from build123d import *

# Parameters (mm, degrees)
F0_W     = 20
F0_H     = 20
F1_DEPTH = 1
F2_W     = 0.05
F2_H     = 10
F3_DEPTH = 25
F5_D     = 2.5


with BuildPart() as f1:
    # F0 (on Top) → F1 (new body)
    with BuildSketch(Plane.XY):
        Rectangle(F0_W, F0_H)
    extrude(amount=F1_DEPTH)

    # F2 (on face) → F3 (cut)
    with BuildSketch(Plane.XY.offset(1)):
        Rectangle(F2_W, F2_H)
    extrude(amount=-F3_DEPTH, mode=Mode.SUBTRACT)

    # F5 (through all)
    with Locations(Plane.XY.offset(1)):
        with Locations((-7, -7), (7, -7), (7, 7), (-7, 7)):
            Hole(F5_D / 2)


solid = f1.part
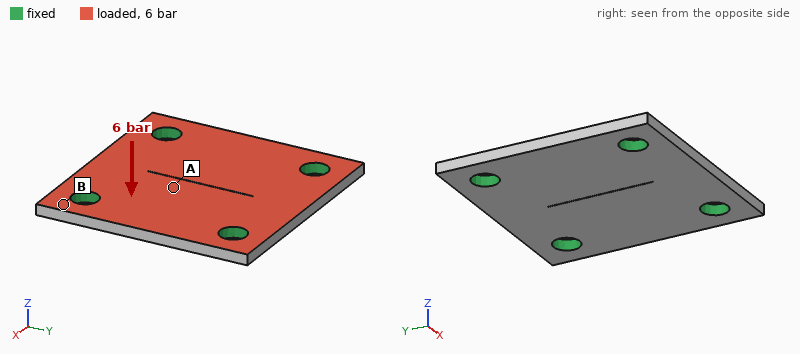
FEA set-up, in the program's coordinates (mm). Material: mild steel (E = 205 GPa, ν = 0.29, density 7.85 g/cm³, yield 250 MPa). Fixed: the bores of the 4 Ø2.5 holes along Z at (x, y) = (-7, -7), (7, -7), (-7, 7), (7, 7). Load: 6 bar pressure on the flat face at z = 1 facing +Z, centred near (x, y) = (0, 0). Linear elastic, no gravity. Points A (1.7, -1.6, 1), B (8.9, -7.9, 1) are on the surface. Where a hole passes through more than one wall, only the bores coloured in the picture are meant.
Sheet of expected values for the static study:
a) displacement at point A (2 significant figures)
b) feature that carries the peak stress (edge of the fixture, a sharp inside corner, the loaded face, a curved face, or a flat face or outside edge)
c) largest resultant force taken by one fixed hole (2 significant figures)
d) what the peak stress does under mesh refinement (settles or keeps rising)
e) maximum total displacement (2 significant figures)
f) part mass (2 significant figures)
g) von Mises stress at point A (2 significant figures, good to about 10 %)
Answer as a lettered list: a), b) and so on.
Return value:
a) 6.4 µm
b) a sharp inside corner
c) 57 N
d) keeps rising
e) 8.4 µm
f) 3.0 g
g) 22 MPa
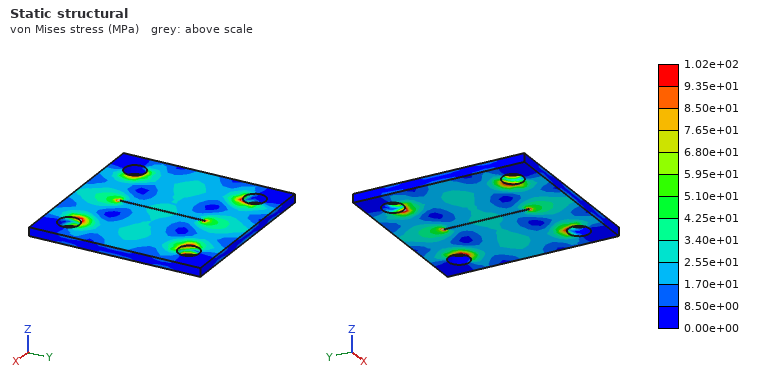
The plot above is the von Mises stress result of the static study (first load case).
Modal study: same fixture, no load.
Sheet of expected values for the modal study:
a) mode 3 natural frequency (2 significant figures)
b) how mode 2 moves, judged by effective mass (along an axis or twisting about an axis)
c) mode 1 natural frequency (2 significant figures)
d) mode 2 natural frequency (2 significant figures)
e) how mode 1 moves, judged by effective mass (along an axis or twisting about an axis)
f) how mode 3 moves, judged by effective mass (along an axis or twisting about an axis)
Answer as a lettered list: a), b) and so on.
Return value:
a) 34 kHz
b) twisting about Y
c) 20 kHz
d) 32 kHz
e) along Z
f) twisting about X
